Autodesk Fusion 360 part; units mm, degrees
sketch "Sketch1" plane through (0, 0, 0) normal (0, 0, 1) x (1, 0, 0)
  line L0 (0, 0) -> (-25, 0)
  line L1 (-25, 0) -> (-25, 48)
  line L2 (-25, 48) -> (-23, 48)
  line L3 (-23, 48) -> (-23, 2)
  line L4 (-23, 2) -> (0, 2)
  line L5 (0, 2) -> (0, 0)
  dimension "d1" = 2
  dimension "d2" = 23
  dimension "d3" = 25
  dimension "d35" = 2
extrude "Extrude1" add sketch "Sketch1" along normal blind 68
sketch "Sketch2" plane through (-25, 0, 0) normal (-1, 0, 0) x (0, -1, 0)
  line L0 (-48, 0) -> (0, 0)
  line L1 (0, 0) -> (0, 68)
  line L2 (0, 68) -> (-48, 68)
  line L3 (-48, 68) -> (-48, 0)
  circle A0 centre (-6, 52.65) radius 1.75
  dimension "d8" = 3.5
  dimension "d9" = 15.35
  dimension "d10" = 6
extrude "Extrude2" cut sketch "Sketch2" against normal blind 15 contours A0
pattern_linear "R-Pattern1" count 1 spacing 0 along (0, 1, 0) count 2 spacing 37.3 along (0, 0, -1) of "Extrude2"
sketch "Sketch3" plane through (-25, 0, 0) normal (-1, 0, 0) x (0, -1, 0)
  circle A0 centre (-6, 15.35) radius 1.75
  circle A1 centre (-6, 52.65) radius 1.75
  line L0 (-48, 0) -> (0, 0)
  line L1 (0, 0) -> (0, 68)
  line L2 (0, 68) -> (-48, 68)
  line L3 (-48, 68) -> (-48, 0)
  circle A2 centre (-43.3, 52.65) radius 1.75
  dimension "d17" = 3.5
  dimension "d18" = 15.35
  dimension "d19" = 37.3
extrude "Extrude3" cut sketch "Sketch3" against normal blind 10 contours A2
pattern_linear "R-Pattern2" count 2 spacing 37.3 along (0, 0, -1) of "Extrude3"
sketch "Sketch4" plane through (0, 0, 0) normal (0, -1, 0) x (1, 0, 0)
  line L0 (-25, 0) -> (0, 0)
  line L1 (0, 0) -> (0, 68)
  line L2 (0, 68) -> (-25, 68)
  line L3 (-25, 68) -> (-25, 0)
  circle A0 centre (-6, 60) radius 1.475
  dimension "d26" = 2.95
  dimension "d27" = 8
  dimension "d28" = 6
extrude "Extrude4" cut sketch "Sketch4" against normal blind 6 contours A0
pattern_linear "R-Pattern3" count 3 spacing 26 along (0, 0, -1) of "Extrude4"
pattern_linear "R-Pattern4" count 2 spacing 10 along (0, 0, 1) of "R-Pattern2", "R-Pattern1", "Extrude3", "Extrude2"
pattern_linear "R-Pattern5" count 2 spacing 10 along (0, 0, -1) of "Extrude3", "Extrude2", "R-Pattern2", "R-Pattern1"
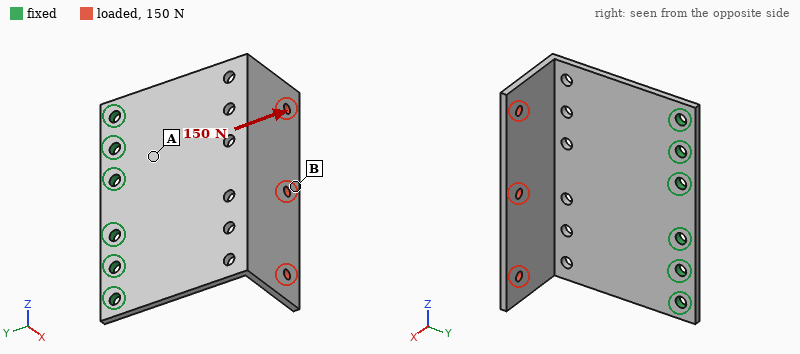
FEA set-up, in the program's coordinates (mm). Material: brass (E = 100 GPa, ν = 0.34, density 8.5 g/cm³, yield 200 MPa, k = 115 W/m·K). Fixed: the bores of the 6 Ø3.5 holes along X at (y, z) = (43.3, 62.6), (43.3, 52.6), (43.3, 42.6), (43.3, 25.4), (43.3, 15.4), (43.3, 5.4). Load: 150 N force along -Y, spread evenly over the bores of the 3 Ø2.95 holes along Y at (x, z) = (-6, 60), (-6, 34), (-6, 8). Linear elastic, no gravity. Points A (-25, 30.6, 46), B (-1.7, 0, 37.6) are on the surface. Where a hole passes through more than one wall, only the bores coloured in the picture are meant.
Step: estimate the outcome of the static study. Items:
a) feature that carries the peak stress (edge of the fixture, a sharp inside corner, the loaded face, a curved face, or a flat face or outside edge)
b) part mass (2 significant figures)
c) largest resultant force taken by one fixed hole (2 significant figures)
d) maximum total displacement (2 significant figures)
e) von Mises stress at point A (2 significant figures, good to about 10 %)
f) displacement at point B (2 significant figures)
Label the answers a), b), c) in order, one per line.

a) a curved face
b) 80 g
c) 29 N
d) 0.83 mm
e) 52 MPa
f) 0.78 mm
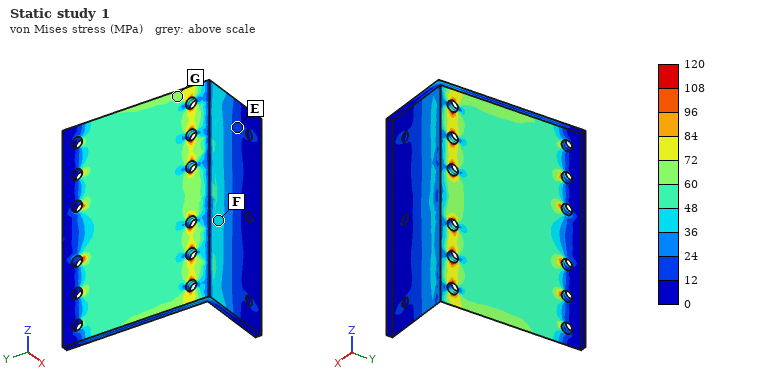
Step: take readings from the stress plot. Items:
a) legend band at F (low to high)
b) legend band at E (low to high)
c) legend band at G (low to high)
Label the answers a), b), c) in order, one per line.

a) 36 to 48 MPa
b) 12 to 24 MPa
c) 60 to 72 MPa
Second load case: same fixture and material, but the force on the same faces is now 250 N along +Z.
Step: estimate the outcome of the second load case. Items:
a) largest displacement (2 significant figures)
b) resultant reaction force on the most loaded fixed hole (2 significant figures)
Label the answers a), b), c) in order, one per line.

a) 0.58 mm
b) 150 N
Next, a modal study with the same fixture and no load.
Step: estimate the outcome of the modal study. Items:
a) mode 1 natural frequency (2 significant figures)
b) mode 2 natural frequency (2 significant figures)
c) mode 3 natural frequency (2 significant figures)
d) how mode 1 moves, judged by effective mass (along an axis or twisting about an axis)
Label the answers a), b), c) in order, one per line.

a) 340 Hz
b) 630 Hz
c) 1200 Hz
d) along X
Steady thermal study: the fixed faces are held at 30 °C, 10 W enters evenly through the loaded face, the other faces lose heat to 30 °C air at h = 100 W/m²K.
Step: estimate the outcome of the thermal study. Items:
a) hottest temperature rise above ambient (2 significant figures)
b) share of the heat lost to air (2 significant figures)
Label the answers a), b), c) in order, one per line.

a) 21 K
b) 73 %
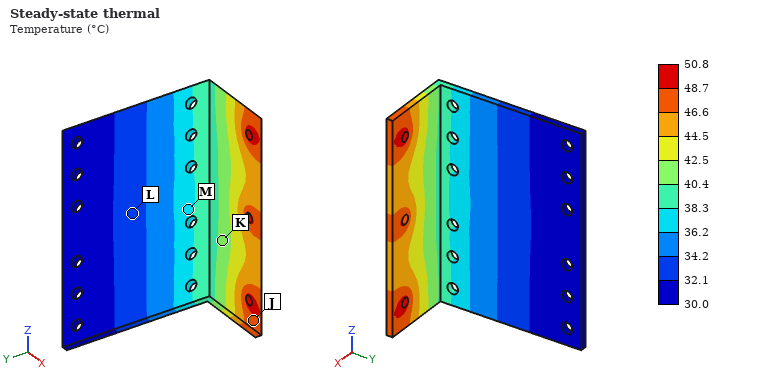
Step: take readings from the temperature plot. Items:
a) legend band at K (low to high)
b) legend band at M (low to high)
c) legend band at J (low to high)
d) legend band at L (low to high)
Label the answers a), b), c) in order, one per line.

a) 40.4 to 42.5 °C
b) 36.2 to 38.3 °C
c) 46.6 to 48.7 °C
d) 32.1 to 34.2 °C
